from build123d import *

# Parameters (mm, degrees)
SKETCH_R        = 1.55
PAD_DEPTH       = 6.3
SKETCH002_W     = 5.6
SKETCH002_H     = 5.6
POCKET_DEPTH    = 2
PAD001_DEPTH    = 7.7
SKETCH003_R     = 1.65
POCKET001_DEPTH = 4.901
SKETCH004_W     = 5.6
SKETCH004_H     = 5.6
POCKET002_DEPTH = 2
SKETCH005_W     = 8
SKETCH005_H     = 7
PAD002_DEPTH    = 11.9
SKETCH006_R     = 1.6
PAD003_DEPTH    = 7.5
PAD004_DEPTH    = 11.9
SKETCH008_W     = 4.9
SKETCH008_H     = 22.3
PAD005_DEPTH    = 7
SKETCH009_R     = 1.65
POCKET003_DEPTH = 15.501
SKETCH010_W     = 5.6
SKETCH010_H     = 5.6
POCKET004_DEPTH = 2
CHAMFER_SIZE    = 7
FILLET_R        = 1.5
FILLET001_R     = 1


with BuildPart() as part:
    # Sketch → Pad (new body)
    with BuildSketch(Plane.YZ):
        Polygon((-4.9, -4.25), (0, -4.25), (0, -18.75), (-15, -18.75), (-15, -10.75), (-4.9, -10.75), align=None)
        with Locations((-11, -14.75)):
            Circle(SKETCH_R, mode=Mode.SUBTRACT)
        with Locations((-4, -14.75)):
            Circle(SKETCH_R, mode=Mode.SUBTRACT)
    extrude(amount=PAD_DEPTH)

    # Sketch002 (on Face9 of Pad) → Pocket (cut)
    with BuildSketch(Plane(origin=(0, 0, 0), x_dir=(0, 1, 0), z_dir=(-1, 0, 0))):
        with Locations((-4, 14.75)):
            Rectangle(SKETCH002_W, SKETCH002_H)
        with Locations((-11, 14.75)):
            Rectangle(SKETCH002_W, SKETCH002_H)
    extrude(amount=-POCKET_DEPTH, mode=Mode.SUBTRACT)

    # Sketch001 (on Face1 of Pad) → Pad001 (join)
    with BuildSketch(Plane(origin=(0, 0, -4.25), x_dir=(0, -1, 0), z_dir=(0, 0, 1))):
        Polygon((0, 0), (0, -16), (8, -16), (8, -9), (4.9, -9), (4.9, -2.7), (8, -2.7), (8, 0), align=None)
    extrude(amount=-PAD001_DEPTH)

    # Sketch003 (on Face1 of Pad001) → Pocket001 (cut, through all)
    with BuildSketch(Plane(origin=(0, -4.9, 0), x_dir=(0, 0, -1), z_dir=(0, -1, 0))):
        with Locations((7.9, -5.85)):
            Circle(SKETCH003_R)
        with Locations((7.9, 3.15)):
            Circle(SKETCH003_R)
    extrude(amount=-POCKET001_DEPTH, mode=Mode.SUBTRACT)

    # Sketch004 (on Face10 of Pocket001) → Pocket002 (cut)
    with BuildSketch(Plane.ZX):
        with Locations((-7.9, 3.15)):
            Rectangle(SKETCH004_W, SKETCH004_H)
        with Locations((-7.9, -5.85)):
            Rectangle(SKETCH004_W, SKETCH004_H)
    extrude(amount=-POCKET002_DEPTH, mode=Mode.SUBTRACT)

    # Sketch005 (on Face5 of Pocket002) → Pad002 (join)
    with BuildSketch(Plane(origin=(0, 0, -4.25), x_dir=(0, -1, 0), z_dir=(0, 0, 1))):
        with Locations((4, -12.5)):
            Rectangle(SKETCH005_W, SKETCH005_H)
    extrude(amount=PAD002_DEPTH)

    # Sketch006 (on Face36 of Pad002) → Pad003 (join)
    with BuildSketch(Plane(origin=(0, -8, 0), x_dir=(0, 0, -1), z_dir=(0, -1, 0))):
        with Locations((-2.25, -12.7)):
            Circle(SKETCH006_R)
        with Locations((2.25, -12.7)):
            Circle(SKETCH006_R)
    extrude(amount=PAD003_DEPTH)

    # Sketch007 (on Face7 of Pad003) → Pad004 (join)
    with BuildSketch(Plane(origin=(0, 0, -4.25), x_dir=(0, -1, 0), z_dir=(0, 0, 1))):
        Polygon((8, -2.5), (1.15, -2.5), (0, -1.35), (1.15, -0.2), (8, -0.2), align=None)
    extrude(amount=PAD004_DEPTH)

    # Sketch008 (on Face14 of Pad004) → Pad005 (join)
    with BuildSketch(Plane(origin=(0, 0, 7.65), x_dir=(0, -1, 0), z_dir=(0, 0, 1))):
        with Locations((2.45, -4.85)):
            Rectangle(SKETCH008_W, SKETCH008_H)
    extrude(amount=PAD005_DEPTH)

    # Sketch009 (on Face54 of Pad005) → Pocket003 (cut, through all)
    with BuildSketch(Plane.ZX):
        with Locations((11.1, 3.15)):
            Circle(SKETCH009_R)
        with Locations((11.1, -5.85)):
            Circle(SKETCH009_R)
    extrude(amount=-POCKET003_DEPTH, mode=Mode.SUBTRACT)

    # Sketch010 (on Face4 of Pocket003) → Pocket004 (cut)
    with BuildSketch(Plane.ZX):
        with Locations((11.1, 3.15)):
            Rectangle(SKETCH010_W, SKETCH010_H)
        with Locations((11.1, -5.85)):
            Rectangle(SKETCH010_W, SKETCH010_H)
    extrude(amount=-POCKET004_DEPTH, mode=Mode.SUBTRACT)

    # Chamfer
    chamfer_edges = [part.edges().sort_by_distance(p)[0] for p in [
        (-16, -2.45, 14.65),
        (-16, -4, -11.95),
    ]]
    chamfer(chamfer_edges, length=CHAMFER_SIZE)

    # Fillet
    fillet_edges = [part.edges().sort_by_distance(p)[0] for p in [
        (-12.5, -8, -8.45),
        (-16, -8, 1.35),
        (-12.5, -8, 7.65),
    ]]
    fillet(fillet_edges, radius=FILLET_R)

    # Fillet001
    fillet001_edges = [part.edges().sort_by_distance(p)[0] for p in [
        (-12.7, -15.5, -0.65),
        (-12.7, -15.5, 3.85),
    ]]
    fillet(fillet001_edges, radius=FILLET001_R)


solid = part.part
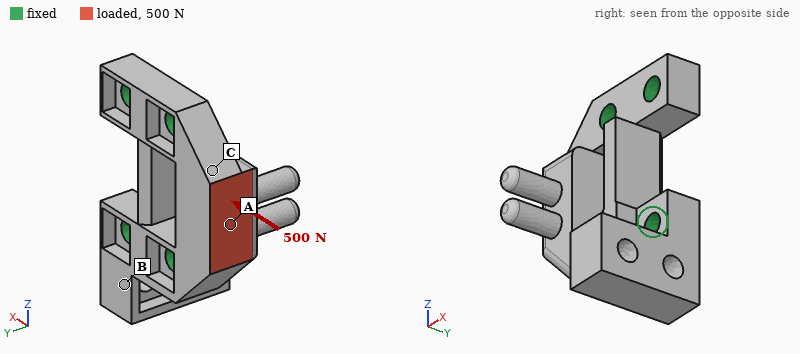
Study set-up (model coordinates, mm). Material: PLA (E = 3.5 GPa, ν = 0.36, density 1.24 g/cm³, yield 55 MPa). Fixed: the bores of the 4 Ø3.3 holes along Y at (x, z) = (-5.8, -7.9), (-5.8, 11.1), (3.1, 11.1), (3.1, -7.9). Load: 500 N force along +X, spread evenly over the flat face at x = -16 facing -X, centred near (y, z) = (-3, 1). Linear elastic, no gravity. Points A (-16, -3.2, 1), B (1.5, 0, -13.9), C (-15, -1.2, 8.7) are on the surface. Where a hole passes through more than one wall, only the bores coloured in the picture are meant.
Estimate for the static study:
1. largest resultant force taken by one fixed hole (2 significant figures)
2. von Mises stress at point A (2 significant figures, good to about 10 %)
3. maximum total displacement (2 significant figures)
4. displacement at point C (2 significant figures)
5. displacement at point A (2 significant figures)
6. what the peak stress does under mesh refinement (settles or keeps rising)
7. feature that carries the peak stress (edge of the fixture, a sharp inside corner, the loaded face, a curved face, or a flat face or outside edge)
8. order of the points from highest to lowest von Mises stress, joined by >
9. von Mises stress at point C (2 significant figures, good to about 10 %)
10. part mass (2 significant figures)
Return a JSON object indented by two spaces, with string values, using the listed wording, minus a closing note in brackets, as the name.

{
  "largest resultant force taken by one fixed hole": "270 N",
  "von Mises stress at point A": "12 MPa",
  "maximum total displacement": "82 µm",
  "displacement at point C": "29 µm",
  "displacement at point A": "58 µm",
  "what the peak stress does under mesh refinement": "keeps rising",
  "feature that carries the peak stress": "a sharp inside corner",
  "order of the points from highest to lowest von Mises stress, joined by >": "A > C > B",
  "von Mises stress at point C": "6.1 MPa",
  "part mass": "3.3 g"
}
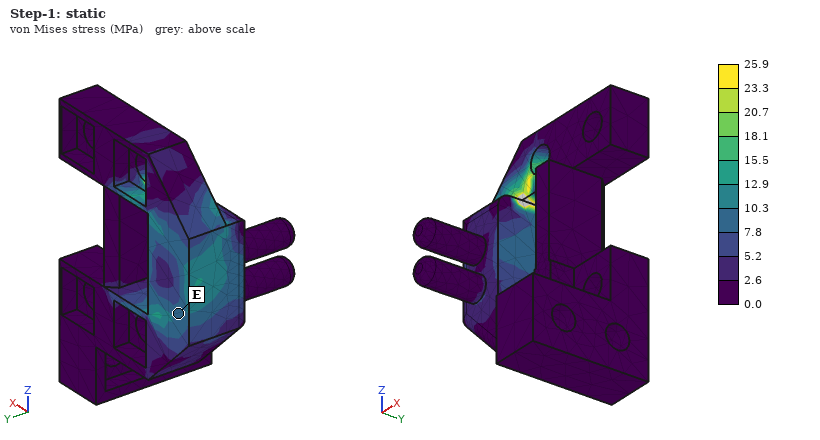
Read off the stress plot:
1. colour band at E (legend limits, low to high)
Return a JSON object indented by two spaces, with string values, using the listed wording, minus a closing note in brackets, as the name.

{
  "colour band at E": "7.8 to 10.3 MPa"
}
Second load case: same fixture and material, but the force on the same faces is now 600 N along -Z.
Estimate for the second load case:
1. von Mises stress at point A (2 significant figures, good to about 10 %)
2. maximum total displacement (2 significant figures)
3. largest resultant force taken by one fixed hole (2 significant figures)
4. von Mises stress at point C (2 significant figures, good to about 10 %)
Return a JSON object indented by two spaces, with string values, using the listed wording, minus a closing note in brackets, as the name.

{
  "von Mises stress at point A": "13 MPa",
  "maximum total displacement": "87 µm",
  "largest resultant force taken by one fixed hole": "400 N",
  "von Mises stress at point C": "8.7 MPa"
}
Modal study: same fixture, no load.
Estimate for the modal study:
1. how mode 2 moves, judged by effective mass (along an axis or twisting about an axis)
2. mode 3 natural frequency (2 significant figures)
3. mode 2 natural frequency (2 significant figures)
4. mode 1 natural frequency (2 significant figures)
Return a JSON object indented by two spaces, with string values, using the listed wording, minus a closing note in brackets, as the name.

{
  "how mode 2 moves, judged by effective mass": "along Y",
  "mode 3 natural frequency": "6100 Hz",
  "mode 2 natural frequency": "4500 Hz",
  "mode 1 natural frequency": "3800 Hz"
}
